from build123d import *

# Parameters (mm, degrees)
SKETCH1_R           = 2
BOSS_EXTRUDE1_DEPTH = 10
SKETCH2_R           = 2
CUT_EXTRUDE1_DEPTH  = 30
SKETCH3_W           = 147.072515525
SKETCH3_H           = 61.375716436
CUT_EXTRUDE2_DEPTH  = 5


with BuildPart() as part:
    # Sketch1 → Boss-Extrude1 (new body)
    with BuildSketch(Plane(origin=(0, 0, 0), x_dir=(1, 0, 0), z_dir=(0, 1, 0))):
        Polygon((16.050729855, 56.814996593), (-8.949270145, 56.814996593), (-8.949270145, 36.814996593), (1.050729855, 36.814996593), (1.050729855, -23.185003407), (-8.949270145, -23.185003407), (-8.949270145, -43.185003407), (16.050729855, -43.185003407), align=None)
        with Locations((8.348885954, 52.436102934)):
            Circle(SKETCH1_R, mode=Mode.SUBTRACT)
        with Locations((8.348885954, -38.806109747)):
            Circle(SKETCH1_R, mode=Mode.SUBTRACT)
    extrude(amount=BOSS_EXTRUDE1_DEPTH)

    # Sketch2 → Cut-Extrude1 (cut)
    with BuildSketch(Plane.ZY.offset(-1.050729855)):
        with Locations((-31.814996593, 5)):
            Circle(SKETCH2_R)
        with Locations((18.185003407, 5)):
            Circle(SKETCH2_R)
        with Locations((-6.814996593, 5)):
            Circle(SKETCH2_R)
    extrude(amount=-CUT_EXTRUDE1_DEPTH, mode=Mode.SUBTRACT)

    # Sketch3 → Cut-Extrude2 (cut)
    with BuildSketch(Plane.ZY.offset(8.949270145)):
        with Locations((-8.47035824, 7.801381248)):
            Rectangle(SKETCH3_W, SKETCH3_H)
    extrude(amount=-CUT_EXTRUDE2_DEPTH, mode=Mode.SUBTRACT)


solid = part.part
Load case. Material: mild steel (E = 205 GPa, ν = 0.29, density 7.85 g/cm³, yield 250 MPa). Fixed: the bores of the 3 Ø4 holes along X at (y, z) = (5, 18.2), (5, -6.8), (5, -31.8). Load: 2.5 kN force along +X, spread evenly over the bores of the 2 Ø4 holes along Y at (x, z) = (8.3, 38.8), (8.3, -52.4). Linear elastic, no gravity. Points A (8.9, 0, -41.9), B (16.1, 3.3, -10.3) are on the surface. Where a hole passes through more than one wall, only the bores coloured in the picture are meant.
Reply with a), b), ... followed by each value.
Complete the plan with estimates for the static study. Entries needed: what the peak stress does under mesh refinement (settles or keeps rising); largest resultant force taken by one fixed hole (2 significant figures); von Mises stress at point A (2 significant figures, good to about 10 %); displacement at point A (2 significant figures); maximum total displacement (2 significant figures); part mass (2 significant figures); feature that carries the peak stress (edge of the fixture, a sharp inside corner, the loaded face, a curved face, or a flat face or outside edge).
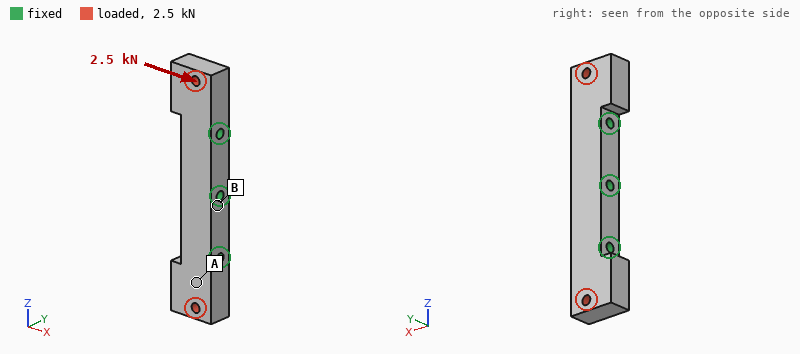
a) keeps rising
b) 1.3 kN
c) 25 MPa
d) 2.7 µm
e) 11 µm
f) 130 g
g) edge of the fixture
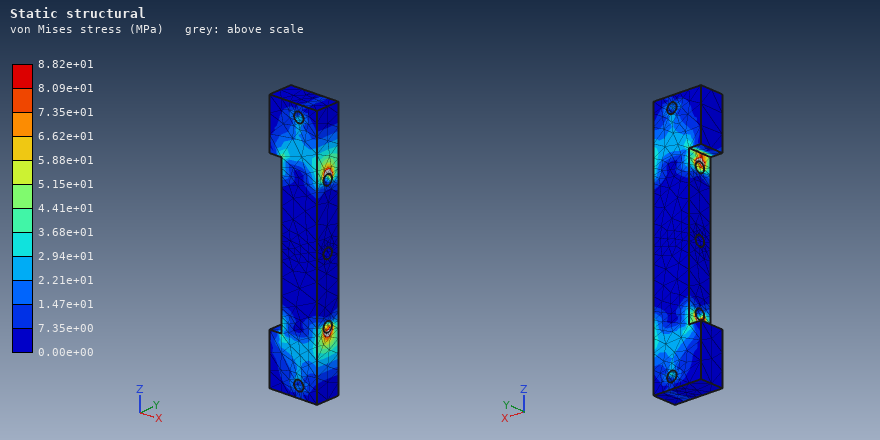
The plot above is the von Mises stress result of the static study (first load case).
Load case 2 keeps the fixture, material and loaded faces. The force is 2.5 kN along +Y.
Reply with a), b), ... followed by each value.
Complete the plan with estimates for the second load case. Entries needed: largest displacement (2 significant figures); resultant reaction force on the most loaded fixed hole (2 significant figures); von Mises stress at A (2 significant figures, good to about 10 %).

a) 25 µm
b) 1.6 kN
c) 47 MPa
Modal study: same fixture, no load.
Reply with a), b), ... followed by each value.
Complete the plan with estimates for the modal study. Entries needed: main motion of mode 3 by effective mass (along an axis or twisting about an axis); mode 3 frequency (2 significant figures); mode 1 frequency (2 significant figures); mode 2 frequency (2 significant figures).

a) along X
b) 15 kHz
c) 9700 Hz
d) 9800 Hz
